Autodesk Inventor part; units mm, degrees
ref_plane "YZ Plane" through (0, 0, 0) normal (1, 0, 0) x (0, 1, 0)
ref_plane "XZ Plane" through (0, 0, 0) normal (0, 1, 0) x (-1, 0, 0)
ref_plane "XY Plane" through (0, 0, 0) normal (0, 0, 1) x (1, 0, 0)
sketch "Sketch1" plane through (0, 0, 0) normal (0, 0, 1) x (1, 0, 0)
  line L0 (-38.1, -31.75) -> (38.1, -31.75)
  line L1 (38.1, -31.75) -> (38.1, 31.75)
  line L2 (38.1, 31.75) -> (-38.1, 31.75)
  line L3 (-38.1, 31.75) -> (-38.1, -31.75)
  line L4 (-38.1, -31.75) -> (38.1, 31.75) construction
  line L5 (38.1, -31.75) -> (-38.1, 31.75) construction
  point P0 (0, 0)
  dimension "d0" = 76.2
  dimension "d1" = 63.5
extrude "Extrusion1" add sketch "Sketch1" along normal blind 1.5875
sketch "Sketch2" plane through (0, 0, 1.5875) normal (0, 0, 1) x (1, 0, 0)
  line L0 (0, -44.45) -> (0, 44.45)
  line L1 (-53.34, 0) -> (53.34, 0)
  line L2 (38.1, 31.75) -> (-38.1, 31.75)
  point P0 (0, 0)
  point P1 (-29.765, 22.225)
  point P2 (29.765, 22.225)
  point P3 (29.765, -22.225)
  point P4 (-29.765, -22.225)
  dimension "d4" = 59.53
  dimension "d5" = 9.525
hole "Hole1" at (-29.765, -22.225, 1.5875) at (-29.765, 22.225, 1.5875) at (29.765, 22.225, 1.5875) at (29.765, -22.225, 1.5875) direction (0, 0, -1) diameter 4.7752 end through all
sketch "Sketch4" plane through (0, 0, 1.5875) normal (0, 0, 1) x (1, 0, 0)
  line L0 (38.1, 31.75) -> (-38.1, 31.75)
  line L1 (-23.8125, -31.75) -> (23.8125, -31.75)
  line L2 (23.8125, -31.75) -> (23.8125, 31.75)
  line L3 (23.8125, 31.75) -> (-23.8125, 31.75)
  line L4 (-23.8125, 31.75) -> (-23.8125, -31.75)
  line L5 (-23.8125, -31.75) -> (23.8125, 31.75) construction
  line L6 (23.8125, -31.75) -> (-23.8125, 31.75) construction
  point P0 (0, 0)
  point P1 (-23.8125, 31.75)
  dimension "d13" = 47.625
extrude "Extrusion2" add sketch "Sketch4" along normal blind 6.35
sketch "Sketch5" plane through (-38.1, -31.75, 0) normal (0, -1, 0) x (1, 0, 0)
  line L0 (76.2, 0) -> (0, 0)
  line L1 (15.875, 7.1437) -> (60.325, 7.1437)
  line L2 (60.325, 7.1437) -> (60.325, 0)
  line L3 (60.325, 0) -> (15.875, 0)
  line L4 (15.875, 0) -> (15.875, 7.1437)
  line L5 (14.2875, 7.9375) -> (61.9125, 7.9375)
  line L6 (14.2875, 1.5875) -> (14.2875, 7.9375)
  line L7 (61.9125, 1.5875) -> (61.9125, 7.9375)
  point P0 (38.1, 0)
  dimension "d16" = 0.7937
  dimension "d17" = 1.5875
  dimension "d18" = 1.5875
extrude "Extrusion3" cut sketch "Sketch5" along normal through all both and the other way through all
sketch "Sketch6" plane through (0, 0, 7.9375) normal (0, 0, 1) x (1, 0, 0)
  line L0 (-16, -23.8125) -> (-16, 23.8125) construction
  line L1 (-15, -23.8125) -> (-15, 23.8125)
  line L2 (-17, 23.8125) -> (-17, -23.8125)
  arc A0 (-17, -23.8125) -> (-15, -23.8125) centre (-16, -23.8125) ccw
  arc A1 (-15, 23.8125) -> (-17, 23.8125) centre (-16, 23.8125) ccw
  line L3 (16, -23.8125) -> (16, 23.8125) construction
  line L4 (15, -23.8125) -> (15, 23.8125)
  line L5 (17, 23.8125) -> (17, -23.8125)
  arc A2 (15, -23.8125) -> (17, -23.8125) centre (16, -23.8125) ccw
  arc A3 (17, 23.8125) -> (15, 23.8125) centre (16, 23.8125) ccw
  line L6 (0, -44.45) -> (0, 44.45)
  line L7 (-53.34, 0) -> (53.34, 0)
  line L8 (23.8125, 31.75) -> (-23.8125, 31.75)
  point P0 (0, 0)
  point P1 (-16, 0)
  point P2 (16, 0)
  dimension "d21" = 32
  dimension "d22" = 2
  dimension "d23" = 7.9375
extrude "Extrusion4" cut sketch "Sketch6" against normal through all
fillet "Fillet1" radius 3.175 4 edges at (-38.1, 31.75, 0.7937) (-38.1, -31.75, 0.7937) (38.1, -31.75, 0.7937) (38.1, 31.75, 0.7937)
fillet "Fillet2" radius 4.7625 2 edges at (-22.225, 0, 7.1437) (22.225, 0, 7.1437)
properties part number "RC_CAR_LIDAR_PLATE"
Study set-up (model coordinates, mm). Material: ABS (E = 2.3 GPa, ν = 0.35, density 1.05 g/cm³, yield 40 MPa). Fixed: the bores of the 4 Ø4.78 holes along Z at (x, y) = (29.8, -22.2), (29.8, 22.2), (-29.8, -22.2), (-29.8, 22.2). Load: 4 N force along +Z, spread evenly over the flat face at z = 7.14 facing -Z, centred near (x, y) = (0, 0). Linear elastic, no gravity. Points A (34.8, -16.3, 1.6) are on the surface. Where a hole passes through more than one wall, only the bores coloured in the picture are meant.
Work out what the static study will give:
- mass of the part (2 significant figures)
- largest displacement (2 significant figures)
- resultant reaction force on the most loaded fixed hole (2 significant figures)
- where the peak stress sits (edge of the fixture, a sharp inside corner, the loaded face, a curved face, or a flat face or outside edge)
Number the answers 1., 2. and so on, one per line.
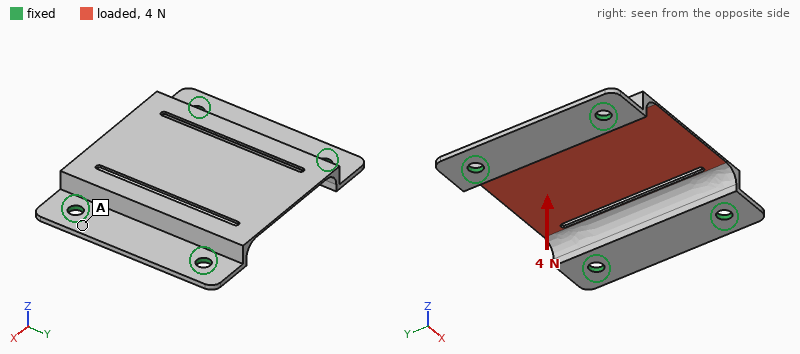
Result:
1. 7.4 g
2. 0.98 mm
3. 2.0 N
4. a curved face
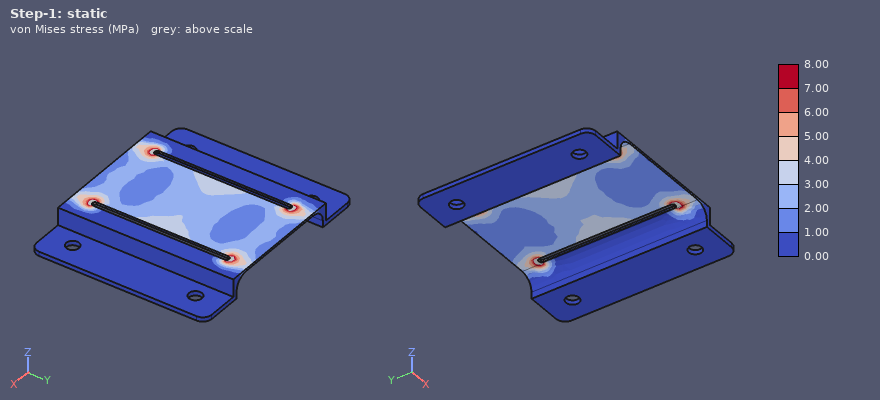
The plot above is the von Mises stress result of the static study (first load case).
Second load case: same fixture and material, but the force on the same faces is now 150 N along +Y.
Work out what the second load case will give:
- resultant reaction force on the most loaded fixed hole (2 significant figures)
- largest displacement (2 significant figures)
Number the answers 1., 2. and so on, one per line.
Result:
1. 41 N
2. 0.30 mm
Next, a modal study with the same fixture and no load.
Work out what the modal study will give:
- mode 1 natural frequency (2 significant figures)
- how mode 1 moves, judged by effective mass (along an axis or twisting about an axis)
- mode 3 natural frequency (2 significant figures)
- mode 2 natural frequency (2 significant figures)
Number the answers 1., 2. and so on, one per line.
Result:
1. 280 Hz
2. along Z
3. 680 Hz
4. 570 Hz
